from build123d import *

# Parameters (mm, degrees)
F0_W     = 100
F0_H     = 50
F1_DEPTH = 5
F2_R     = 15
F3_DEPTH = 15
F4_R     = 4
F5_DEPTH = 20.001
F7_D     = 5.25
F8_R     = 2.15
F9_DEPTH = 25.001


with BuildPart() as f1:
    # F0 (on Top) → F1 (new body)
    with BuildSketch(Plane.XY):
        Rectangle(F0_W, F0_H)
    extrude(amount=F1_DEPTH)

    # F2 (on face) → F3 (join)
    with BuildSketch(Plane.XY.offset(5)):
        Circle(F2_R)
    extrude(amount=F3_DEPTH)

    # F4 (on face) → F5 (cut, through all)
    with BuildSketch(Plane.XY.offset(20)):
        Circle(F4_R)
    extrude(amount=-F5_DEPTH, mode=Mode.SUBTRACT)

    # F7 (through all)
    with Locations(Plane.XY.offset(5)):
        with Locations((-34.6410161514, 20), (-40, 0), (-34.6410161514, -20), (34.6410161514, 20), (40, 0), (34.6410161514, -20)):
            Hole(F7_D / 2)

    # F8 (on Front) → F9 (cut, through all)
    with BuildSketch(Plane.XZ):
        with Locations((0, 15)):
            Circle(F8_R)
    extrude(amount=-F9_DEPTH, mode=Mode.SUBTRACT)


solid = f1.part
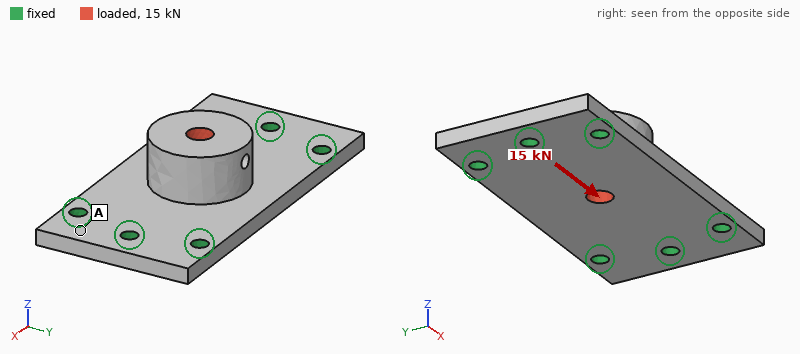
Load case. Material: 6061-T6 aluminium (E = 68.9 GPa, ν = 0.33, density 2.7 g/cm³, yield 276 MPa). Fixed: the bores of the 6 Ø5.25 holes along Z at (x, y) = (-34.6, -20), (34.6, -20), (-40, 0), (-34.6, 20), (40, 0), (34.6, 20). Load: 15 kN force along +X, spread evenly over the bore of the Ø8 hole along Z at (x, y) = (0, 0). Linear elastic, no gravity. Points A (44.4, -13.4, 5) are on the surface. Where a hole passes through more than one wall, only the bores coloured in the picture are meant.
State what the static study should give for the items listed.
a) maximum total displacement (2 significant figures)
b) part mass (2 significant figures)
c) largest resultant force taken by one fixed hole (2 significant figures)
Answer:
0.11 mm
91 g
2.7 kN
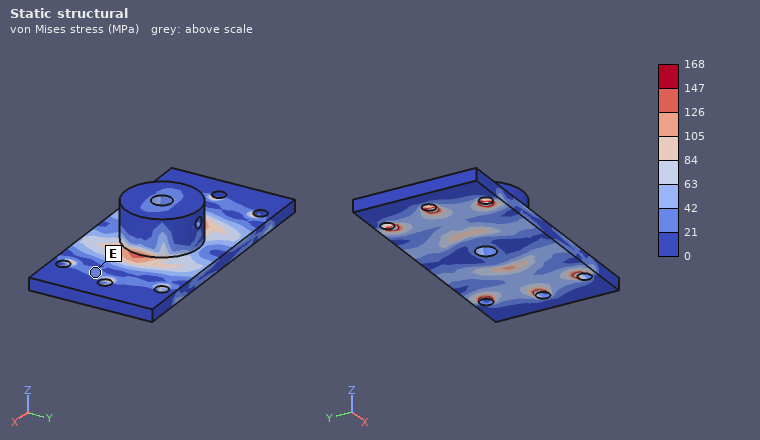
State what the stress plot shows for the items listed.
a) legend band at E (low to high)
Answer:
21 to 42 MPa
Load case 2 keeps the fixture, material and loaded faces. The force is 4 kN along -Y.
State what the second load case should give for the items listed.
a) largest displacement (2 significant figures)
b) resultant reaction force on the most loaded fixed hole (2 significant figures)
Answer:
72 µm
1.2 kN
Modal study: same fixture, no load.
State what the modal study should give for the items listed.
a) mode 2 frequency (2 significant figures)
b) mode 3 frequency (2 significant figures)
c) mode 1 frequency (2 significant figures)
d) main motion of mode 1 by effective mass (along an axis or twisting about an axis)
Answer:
5500 Hz
9100 Hz
4500 Hz
along Z
